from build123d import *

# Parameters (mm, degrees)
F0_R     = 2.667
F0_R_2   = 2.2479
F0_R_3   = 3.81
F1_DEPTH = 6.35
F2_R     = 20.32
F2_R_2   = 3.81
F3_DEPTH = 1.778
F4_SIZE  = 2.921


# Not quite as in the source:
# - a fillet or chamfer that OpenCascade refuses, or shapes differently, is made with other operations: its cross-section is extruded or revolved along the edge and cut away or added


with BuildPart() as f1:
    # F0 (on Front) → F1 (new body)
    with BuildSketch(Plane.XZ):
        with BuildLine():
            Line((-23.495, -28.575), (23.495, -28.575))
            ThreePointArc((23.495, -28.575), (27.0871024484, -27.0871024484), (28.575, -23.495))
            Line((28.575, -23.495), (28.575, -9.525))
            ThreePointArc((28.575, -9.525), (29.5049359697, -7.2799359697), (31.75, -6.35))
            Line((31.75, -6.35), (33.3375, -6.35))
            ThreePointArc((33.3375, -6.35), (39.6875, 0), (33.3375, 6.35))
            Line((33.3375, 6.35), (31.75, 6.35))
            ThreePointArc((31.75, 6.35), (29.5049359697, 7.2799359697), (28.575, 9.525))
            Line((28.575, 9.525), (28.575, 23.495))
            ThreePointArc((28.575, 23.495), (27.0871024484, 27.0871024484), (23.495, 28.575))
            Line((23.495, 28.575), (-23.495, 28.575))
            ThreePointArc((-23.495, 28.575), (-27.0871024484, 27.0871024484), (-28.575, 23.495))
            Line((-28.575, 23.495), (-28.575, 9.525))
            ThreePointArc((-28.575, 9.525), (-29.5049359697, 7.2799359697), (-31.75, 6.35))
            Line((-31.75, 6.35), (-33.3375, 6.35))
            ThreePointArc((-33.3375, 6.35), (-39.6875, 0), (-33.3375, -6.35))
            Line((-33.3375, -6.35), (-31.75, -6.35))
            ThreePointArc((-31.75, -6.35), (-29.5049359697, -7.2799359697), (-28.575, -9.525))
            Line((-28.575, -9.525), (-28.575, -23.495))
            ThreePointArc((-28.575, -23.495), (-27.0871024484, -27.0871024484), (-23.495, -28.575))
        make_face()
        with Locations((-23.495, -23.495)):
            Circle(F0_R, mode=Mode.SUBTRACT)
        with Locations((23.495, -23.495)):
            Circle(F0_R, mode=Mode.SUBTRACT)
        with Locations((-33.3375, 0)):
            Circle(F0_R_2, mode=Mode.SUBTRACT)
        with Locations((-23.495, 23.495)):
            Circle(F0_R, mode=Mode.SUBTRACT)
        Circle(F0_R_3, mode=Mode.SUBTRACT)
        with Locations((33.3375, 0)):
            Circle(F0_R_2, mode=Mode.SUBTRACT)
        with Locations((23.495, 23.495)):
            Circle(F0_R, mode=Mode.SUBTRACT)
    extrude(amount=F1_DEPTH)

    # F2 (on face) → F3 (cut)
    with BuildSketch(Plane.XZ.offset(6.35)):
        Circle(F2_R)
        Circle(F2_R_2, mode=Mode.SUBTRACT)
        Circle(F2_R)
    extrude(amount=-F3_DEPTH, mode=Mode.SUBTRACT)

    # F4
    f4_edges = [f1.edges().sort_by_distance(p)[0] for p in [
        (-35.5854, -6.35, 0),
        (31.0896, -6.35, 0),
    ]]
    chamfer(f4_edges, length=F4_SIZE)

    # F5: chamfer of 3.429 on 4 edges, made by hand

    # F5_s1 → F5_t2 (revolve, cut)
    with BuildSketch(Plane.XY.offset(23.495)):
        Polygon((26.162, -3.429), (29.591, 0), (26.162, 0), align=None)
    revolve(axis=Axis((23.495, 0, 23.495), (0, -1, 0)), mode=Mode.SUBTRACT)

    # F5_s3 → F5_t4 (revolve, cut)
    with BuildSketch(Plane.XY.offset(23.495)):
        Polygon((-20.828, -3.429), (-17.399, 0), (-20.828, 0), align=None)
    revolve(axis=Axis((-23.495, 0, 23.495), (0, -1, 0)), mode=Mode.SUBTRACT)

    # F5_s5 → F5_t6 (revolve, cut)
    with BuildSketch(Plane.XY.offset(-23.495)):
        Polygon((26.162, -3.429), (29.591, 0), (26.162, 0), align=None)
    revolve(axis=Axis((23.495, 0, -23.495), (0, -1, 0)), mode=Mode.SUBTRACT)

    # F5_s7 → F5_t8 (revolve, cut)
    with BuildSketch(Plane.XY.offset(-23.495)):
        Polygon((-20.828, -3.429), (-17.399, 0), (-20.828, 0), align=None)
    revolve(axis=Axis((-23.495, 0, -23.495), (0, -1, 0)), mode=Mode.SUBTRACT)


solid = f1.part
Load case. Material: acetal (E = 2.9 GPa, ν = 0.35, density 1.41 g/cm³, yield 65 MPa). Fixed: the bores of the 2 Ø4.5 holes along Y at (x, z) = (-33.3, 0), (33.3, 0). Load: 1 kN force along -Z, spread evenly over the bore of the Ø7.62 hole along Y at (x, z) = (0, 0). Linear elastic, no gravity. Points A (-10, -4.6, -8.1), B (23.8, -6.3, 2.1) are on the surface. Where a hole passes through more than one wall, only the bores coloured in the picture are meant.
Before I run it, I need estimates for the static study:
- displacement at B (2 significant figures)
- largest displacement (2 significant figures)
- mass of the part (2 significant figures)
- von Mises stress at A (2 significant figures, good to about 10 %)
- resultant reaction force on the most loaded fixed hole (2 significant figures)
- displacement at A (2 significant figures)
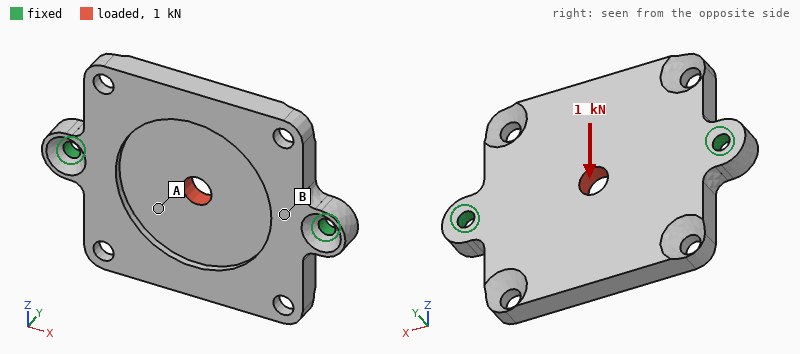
0.064 mm
0.14 mm
26 g
4.5 MPa
500 N
0.10 mm
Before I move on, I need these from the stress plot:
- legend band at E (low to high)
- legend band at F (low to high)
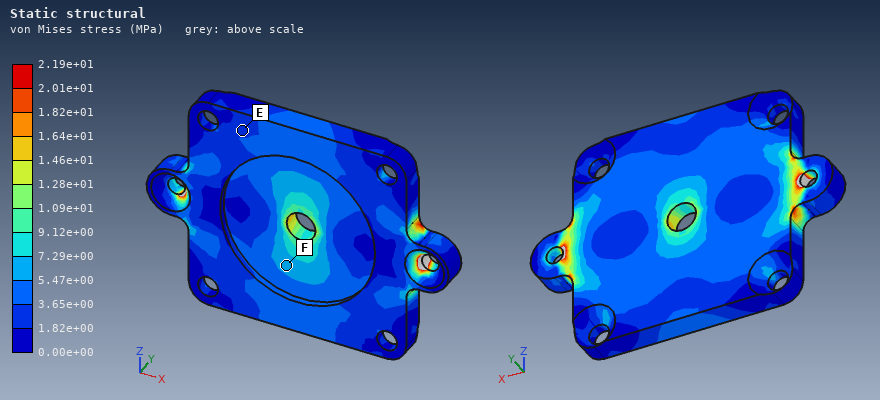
1.82e+00 to 3.65e+00 MPa
5.47e+00 to 7.29e+00 MPa
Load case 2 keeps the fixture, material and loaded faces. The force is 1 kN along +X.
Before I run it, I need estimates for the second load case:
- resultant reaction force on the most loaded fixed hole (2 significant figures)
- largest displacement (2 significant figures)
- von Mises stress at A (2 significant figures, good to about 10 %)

500 N
73 µm
3.8 MPa
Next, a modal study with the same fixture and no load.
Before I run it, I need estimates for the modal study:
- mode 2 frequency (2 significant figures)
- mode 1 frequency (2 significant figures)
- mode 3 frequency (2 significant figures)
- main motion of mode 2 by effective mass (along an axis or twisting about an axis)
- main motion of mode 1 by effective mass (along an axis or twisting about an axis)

960 Hz
670 Hz
2000 Hz
along Y
twisting about X
